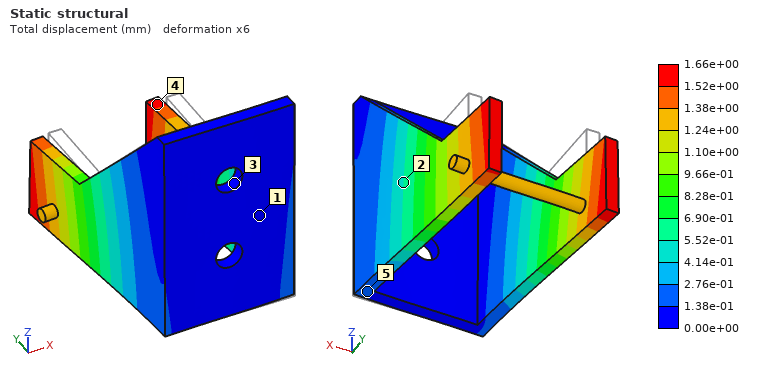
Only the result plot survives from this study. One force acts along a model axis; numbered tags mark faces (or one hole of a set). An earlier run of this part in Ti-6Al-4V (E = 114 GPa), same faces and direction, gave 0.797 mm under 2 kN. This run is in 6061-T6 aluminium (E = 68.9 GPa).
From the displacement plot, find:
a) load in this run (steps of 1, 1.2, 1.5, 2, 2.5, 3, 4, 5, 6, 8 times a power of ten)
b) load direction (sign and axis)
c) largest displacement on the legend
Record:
2.5 kN
-X
1.66e+00 mm
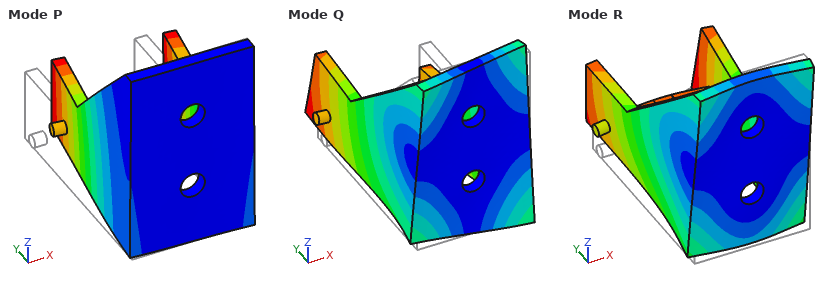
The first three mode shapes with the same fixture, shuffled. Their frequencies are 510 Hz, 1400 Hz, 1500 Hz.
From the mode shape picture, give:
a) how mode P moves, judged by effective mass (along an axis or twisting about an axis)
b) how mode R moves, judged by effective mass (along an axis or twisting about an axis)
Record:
along X
along Z
